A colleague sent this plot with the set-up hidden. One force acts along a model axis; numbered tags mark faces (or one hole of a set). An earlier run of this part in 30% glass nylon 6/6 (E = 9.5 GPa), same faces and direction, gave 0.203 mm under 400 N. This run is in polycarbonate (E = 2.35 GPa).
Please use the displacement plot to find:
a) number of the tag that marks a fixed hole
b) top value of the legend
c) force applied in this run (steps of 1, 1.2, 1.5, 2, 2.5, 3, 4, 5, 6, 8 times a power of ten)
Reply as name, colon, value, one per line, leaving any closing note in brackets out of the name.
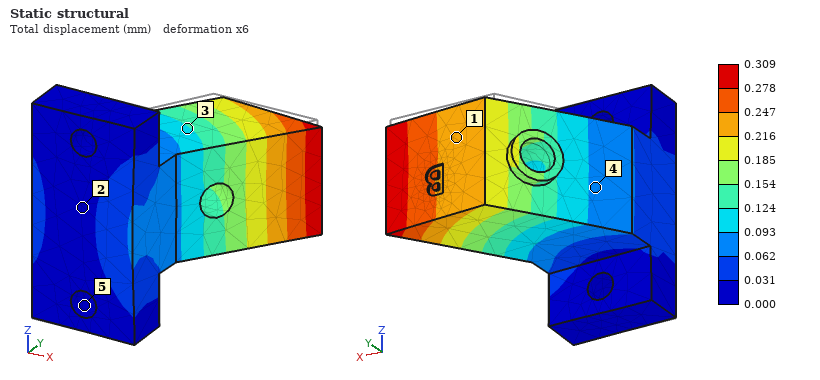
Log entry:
number of the tag that marks a fixed hole: 5
top value of the legend: 0.309 mm
force applied in this run: 150 N
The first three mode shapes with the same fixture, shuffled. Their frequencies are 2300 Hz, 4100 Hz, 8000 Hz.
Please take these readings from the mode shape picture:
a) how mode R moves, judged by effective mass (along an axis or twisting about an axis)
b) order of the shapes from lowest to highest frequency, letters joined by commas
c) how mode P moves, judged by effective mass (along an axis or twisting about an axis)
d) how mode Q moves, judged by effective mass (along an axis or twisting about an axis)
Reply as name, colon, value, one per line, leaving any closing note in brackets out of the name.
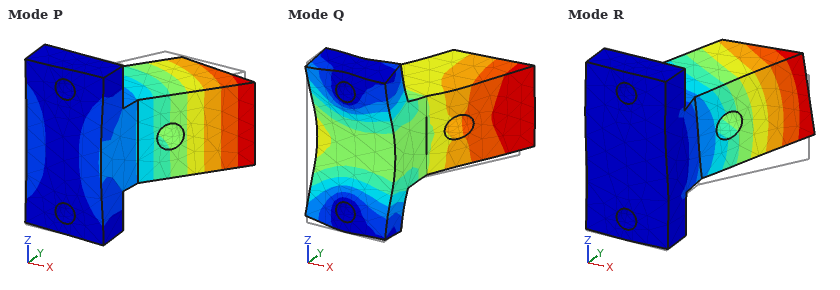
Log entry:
how mode R moves, judged by effective mass: along Z
order of the shapes from lowest to highest frequency, letters joined by commas: P, R, Q
how mode P moves, judged by effective mass: along X
how mode Q moves, judged by effective mass: along Y
